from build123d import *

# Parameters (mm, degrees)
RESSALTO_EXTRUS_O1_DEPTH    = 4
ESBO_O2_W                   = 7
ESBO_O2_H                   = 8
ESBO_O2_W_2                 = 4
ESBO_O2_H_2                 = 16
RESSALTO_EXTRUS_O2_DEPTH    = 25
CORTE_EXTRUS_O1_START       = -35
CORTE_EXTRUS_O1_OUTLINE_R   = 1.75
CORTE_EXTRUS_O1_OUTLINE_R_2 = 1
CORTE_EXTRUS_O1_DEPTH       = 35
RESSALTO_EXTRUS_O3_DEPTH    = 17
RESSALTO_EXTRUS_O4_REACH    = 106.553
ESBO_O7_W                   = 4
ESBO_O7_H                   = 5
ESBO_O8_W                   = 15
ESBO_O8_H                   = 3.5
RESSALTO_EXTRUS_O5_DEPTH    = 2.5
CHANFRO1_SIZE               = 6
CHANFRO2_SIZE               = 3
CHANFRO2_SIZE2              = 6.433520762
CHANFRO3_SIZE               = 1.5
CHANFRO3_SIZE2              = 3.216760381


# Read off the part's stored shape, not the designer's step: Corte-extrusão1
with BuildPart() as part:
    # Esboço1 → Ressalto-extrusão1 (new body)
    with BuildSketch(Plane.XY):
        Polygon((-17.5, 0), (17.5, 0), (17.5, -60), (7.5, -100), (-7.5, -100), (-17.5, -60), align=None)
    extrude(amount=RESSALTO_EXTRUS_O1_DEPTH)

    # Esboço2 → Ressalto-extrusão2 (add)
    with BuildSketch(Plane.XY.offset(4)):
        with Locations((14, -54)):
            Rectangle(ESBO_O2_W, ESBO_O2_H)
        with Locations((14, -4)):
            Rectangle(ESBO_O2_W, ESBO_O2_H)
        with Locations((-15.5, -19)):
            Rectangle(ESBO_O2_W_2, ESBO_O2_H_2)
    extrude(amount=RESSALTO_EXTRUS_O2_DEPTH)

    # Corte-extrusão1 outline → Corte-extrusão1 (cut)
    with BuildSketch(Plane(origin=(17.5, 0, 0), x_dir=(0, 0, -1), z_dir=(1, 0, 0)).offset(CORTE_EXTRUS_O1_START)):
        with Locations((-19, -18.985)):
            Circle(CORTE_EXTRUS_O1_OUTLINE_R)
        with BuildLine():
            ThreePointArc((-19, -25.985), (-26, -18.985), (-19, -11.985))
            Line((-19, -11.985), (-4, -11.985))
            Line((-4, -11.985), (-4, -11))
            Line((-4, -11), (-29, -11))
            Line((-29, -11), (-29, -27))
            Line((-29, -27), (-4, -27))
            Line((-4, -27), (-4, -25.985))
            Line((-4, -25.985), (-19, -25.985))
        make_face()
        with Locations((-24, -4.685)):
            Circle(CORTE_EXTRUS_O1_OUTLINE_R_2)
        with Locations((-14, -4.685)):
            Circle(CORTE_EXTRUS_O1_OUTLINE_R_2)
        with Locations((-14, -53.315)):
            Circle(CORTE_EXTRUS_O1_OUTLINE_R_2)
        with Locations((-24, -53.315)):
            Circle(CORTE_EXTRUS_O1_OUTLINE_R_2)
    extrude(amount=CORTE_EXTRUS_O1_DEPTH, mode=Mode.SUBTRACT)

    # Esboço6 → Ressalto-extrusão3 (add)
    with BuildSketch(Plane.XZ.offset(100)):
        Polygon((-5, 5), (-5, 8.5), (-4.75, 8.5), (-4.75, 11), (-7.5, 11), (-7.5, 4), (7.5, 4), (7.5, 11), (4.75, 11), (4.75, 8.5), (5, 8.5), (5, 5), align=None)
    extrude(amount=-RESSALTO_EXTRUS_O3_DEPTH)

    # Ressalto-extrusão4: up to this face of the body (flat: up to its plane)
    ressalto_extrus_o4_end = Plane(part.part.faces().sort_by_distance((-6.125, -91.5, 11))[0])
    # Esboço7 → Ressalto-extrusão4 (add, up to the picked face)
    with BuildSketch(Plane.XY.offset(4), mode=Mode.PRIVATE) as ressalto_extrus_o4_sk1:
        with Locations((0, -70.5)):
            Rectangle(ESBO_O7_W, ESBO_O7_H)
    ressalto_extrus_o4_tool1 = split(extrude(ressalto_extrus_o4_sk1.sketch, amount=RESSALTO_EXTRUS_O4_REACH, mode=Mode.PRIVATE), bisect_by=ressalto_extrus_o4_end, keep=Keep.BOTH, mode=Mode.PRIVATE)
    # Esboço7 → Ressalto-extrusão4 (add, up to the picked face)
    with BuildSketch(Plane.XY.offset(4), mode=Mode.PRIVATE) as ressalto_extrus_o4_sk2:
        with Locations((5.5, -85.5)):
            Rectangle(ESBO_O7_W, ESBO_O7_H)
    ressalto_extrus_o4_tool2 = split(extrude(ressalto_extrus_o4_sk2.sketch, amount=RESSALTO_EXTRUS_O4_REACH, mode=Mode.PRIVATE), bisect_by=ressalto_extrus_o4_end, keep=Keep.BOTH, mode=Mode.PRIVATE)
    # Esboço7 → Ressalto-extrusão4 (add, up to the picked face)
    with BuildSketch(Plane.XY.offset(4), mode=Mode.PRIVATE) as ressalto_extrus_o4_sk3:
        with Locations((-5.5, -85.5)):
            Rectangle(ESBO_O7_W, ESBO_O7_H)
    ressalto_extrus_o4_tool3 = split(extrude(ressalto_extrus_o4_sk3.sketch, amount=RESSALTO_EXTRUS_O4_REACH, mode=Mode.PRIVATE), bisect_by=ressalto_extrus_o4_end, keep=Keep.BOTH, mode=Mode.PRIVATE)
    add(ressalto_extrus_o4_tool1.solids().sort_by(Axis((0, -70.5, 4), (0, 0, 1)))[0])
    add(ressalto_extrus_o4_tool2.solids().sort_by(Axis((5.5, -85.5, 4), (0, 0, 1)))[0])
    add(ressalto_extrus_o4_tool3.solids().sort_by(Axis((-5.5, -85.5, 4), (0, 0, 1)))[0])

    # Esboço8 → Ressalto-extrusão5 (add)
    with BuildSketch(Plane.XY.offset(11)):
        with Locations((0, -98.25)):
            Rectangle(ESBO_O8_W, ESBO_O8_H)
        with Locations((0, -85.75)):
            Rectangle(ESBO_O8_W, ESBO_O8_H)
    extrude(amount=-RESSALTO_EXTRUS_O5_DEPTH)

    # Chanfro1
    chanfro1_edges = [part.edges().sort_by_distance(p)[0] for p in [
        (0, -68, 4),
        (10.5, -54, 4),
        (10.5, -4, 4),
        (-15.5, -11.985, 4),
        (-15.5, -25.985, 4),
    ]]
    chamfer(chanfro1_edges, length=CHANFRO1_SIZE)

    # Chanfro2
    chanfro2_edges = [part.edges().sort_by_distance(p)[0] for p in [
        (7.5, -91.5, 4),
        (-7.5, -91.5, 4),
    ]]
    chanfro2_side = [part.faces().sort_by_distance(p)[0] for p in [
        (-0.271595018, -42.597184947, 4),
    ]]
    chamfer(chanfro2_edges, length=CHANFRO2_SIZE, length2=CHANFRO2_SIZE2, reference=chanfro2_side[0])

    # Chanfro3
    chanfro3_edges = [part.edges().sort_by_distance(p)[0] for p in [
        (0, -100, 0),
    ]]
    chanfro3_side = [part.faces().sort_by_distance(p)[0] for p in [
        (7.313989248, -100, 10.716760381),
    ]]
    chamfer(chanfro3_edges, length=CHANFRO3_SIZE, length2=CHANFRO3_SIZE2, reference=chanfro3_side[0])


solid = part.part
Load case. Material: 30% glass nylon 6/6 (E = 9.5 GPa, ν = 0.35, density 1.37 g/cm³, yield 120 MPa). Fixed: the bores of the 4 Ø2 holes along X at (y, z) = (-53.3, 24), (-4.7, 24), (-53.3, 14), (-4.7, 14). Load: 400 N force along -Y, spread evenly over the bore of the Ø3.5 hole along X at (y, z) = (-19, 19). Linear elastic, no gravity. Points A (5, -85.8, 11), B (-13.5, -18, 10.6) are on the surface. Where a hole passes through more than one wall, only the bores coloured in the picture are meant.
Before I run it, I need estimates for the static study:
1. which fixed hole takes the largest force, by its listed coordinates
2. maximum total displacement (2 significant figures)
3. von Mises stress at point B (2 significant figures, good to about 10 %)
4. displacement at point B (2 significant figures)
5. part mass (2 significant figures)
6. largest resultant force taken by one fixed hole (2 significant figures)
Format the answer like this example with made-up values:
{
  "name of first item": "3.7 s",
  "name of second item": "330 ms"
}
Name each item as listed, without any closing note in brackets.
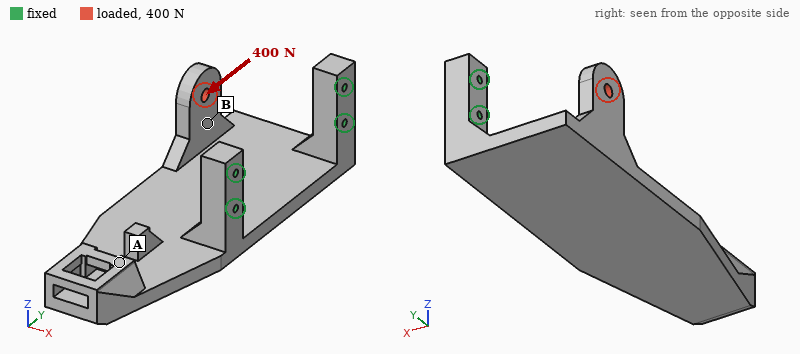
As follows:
{
  "which fixed hole takes the largest force, by its listed coordinates": "(-4.7, 14)",
  "maximum total displacement": "1.2 mm",
  "von Mises stress at point B": "21 MPa",
  "displacement at point B": "0.56 mm",
  "part mass": "25 g",
  "largest resultant force taken by one fixed hole": "470 N"
}
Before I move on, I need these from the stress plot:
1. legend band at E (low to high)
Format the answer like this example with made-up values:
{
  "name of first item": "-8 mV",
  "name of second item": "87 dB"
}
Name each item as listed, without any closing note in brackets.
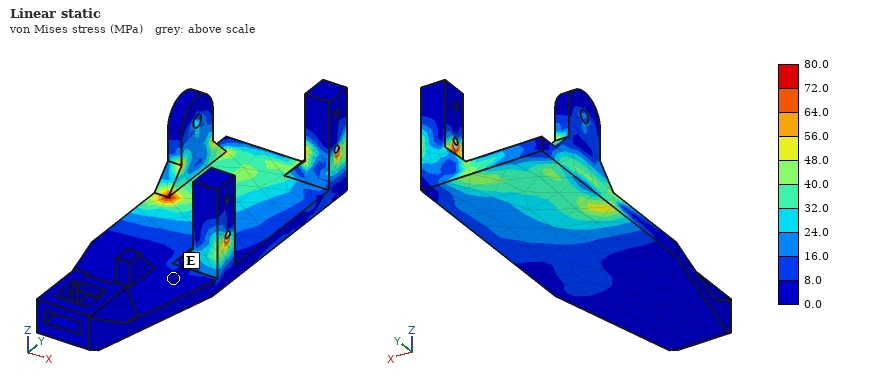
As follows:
{
  "legend band at E": "0.0 to 8.0 MPa"
}
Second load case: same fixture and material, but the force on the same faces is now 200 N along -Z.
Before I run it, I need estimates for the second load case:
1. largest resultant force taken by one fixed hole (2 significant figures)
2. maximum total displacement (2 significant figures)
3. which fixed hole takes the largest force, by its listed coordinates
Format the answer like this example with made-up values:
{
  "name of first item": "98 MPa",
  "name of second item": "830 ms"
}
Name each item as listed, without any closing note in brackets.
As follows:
{
  "largest resultant force taken by one fixed hole": "150 N",
  "maximum total displacement": "1.2 mm",
  "which fixed hole takes the largest force, by its listed coordinates": "(-4.7, 14)"
}
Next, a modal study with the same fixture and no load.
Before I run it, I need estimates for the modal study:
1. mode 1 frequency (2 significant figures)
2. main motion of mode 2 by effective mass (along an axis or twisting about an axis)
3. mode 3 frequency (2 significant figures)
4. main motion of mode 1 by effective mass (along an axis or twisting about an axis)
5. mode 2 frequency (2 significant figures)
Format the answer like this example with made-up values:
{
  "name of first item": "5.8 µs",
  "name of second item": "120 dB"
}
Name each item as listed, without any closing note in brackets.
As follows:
{
  "mode 1 frequency": "650 Hz",
  "main motion of mode 2 by effective mass": "along Z",
  "mode 3 frequency": "1600 Hz",
  "main motion of mode 1 by effective mass": "along Z",
  "mode 2 frequency": "1000 Hz"
}
